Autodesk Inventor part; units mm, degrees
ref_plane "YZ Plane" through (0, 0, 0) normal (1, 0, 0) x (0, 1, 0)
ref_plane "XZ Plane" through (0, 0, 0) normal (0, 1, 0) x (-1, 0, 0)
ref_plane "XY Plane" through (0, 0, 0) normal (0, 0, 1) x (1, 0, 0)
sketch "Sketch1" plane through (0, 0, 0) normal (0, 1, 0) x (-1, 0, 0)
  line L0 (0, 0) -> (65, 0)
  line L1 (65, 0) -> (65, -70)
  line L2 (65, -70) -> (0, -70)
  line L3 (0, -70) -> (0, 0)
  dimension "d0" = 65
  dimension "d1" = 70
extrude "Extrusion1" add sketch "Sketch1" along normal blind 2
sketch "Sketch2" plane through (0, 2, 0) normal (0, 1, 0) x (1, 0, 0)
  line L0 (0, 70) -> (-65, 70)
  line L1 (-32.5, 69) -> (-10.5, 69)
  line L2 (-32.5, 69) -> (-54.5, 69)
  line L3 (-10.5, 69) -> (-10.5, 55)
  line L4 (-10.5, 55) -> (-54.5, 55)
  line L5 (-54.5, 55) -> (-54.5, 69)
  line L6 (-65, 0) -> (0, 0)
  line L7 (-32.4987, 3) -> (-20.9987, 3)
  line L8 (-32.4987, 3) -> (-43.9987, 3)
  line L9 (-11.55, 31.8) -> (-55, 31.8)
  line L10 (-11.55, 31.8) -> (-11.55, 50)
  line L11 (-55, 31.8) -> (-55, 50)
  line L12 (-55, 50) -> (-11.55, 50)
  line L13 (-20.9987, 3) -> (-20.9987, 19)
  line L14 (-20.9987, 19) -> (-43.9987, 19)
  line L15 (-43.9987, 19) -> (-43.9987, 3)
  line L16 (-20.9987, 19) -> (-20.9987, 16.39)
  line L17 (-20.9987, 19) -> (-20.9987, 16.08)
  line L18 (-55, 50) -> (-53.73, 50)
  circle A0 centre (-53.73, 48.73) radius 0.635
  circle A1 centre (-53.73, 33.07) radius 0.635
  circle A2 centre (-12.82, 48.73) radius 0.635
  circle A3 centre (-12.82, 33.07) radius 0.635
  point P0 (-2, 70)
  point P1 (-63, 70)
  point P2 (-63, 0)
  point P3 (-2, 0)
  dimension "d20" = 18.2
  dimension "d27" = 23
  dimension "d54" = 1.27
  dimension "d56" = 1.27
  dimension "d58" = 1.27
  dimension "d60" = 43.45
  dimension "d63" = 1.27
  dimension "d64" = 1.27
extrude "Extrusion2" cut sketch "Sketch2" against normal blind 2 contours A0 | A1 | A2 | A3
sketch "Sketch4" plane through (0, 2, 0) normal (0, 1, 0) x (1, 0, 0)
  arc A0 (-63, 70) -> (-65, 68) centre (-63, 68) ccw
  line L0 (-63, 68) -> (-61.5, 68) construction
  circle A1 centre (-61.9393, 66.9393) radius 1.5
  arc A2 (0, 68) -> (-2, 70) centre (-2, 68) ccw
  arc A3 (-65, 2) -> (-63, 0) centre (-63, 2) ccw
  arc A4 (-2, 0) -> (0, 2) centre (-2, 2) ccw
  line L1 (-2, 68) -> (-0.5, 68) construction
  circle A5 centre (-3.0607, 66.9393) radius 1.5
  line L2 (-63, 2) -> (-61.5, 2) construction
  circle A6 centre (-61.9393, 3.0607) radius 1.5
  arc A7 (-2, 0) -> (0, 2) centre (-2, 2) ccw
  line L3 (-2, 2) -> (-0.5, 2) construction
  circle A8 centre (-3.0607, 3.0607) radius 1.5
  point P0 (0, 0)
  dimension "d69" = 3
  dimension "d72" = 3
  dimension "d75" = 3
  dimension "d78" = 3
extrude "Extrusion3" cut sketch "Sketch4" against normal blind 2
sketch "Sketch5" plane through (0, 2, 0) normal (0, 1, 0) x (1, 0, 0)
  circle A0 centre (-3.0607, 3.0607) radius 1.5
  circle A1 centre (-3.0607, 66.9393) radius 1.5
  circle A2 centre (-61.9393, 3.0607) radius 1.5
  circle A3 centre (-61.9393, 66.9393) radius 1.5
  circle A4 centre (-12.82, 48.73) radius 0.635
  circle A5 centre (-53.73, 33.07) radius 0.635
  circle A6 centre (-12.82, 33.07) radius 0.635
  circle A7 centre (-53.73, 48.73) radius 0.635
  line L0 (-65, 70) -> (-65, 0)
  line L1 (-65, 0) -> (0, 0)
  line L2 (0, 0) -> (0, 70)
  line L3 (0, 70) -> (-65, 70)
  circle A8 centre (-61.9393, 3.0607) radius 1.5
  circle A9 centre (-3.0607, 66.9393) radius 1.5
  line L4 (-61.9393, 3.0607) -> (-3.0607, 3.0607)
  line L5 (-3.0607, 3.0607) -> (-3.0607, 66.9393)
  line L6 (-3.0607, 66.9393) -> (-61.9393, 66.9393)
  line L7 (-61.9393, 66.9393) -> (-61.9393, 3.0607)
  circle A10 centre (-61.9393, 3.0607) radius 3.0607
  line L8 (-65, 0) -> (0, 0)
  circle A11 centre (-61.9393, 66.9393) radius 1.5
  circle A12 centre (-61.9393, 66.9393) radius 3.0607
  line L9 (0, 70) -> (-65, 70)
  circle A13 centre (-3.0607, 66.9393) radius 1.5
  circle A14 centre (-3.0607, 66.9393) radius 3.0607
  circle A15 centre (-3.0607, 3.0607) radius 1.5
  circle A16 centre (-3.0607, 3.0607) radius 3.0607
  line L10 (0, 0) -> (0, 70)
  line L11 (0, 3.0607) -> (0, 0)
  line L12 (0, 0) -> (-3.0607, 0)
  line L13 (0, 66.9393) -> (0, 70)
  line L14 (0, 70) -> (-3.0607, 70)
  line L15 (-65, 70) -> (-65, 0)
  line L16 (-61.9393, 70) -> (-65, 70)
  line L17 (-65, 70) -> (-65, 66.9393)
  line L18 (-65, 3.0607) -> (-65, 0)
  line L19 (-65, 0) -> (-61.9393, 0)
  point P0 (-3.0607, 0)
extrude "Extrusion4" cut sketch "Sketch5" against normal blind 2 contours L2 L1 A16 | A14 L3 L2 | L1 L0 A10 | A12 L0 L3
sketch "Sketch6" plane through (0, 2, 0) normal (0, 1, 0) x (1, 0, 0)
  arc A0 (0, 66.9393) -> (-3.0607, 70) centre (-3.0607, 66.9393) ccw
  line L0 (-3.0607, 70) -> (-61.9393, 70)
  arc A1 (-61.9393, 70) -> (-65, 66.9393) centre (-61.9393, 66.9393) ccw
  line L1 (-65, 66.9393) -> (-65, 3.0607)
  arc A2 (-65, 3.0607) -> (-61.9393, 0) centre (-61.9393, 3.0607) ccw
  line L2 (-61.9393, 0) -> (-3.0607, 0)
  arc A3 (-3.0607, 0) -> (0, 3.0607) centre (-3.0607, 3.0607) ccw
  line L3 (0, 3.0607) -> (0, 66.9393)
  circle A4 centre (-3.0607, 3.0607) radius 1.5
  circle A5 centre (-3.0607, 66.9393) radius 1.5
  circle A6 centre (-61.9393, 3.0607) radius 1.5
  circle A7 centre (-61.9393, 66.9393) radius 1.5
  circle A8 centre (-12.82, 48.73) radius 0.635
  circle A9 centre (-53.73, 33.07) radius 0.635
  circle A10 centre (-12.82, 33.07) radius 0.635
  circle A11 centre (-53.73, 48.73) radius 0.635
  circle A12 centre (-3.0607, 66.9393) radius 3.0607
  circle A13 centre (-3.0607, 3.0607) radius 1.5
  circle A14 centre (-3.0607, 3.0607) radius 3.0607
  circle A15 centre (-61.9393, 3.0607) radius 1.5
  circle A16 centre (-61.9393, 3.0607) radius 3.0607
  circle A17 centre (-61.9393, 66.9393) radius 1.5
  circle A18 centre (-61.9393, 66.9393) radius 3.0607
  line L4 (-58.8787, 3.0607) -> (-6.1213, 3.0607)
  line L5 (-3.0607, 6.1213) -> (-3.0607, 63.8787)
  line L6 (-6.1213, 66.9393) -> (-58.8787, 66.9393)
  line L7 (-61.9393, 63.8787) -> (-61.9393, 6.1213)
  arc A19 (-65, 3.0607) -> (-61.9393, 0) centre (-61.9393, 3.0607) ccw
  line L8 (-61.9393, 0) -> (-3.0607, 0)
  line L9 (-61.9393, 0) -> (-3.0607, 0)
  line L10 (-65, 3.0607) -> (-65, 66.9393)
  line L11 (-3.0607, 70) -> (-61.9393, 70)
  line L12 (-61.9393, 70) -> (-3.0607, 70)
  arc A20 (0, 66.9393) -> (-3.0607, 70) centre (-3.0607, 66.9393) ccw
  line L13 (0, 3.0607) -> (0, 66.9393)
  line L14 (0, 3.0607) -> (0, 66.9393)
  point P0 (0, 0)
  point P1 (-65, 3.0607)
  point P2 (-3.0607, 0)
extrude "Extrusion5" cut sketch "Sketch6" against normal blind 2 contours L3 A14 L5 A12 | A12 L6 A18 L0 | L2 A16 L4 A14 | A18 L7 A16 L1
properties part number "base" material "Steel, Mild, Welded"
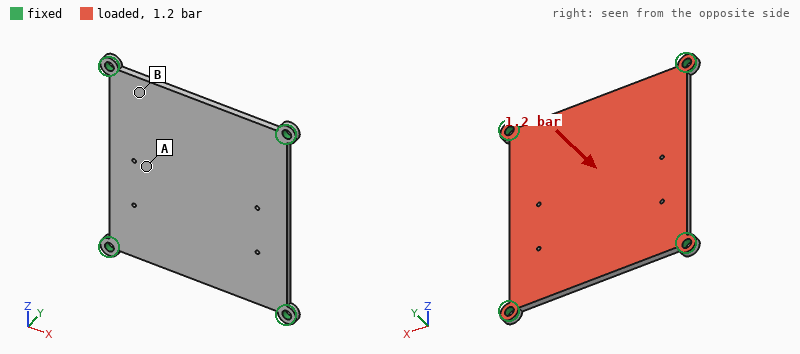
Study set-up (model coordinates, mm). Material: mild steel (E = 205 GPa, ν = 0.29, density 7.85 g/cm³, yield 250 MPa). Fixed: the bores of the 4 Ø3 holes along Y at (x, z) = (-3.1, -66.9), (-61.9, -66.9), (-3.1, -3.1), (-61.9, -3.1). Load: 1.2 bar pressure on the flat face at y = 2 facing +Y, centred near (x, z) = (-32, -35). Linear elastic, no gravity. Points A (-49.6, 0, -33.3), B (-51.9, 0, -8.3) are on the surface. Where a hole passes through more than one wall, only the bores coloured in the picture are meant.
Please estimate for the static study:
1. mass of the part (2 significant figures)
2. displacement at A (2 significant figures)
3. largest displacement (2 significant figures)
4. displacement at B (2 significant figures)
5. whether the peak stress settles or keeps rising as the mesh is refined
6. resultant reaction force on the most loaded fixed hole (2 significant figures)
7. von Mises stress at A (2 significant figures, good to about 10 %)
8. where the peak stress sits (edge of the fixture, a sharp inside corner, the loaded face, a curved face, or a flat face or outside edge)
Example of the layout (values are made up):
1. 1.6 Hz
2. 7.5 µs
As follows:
1. 60 g
2. 0.099 mm
3. 0.12 mm
4. 0.033 mm
5. keeps rising
6. 110 N
7. 45 MPa
8. edge of the fixture
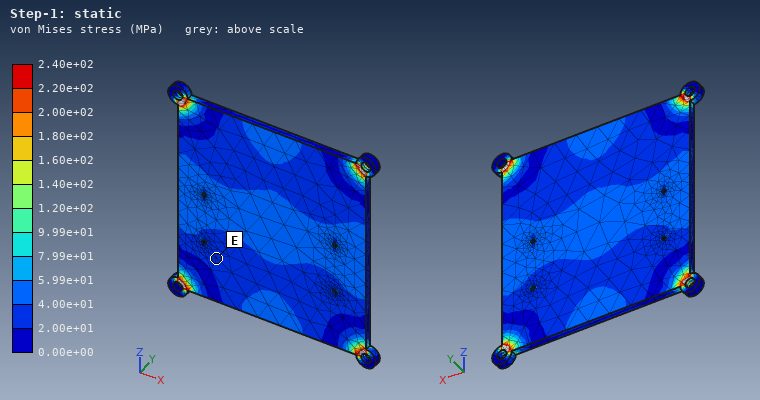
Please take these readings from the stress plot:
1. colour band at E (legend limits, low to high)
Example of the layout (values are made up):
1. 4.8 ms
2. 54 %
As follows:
1. 2.00e+01 to 4.00e+01 MPa
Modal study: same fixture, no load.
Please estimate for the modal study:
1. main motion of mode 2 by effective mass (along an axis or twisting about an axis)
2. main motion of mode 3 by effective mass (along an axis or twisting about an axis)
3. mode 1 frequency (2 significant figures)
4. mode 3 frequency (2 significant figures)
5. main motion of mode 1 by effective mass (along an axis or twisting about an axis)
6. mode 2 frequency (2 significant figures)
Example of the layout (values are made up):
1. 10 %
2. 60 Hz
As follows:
1. twisting about Z
2. twisting about X
3. 1500 Hz
4. 3100 Hz
5. along Y
6. 2900 Hz
